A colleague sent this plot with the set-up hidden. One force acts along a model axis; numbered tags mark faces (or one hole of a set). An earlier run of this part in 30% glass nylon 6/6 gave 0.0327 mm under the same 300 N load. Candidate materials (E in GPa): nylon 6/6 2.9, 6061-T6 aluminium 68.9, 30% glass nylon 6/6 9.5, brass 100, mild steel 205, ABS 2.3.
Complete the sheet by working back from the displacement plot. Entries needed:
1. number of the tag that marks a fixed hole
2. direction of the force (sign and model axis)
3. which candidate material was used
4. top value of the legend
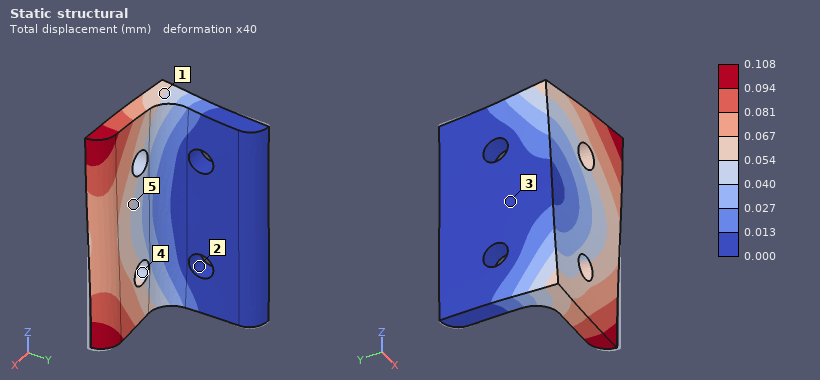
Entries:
2
+Z
nylon 6/6
0.108 mm
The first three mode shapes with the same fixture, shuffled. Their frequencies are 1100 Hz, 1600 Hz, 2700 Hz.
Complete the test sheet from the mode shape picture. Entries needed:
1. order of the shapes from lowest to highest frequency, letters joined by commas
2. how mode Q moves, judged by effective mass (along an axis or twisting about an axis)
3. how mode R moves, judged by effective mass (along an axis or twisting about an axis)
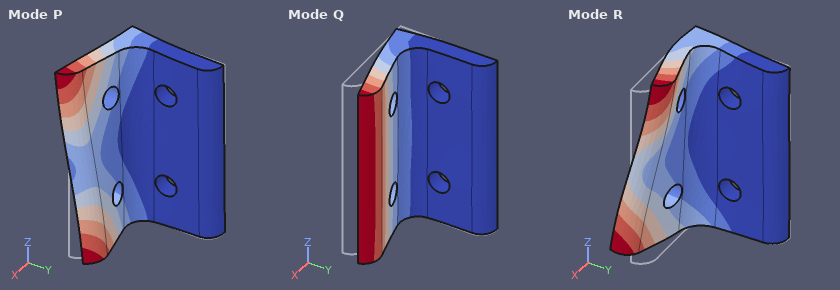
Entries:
Q, P, R
along Y
along Z
